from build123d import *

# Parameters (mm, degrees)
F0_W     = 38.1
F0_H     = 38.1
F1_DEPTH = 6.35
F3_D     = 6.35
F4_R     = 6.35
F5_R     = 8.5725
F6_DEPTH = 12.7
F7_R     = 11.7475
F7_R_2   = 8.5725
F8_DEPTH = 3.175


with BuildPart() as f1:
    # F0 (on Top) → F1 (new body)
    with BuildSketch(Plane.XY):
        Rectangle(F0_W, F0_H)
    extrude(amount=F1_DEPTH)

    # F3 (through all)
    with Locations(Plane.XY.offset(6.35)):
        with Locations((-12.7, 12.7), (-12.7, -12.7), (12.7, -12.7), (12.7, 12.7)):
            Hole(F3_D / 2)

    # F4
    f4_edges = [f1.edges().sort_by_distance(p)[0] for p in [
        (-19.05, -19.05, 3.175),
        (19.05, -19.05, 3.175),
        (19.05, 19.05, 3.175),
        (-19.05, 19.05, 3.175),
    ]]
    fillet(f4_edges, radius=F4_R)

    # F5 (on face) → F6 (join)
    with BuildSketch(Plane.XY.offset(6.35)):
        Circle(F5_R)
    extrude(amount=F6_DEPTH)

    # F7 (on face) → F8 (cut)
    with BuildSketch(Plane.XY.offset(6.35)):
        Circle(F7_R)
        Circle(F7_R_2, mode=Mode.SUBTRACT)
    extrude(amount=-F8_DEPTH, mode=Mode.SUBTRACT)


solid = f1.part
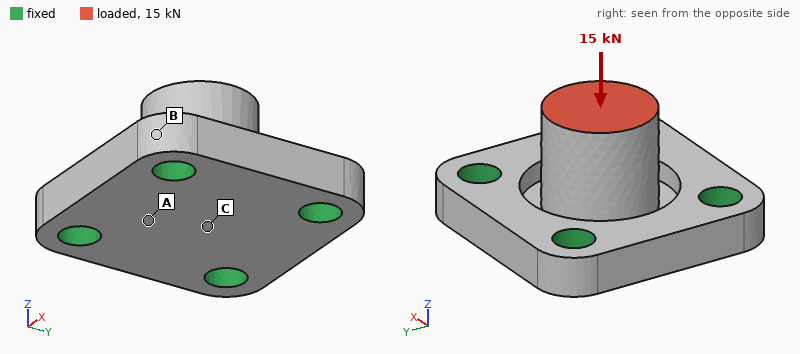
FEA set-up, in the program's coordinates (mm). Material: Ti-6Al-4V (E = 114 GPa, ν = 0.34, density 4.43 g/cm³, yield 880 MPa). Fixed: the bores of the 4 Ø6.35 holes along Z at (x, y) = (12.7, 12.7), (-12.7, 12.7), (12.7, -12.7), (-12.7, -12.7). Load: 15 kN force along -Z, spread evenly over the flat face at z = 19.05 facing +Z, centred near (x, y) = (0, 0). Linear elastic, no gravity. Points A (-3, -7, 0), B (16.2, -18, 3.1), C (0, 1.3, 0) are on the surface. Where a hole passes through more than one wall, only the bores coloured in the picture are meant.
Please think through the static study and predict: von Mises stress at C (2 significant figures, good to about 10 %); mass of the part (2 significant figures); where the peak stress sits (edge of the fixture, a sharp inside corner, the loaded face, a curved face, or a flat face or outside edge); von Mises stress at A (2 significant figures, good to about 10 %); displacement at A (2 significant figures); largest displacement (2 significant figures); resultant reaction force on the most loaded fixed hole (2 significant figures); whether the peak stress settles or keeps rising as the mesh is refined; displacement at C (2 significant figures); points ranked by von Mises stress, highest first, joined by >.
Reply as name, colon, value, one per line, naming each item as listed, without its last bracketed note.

von Mises stress at C: 110 MPa
mass of the part: 46 g
where the peak stress sits: edge of the fixture
von Mises stress at A: 190 MPa
displacement at A: 34 µm
largest displacement: 46 µm
resultant reaction force on the most loaded fixed hole: 3.8 kN
whether the peak stress settles or keeps rising as the mesh is refined: keeps rising
displacement at C: 40 µm
points ranked by von Mises stress, highest first, joined by >: A > C > B
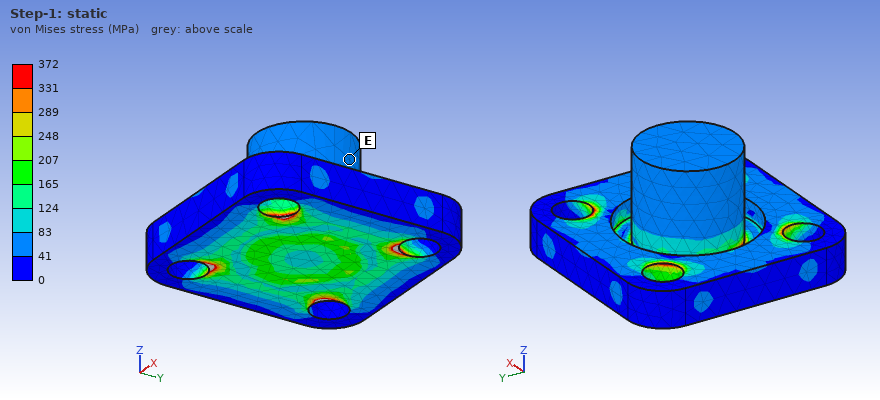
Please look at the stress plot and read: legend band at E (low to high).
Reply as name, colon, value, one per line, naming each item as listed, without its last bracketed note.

legend band at E: 41 to 83 MPa
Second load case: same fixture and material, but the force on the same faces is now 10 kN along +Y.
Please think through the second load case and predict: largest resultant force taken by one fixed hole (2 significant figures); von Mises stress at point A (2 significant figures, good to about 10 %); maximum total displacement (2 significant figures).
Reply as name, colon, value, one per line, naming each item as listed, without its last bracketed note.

largest resultant force taken by one fixed hole: 5.3 kN
von Mises stress at point A: 410 MPa
maximum total displacement: 0.18 mm
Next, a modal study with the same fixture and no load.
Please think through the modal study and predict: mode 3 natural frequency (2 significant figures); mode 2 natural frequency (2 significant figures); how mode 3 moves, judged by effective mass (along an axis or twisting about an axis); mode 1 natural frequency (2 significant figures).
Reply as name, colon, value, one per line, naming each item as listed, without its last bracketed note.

mode 3 natural frequency: 21 kHz
mode 2 natural frequency: 15 kHz
how mode 3 moves, judged by effective mass: along Z
mode 1 natural frequency: 15 kHz
